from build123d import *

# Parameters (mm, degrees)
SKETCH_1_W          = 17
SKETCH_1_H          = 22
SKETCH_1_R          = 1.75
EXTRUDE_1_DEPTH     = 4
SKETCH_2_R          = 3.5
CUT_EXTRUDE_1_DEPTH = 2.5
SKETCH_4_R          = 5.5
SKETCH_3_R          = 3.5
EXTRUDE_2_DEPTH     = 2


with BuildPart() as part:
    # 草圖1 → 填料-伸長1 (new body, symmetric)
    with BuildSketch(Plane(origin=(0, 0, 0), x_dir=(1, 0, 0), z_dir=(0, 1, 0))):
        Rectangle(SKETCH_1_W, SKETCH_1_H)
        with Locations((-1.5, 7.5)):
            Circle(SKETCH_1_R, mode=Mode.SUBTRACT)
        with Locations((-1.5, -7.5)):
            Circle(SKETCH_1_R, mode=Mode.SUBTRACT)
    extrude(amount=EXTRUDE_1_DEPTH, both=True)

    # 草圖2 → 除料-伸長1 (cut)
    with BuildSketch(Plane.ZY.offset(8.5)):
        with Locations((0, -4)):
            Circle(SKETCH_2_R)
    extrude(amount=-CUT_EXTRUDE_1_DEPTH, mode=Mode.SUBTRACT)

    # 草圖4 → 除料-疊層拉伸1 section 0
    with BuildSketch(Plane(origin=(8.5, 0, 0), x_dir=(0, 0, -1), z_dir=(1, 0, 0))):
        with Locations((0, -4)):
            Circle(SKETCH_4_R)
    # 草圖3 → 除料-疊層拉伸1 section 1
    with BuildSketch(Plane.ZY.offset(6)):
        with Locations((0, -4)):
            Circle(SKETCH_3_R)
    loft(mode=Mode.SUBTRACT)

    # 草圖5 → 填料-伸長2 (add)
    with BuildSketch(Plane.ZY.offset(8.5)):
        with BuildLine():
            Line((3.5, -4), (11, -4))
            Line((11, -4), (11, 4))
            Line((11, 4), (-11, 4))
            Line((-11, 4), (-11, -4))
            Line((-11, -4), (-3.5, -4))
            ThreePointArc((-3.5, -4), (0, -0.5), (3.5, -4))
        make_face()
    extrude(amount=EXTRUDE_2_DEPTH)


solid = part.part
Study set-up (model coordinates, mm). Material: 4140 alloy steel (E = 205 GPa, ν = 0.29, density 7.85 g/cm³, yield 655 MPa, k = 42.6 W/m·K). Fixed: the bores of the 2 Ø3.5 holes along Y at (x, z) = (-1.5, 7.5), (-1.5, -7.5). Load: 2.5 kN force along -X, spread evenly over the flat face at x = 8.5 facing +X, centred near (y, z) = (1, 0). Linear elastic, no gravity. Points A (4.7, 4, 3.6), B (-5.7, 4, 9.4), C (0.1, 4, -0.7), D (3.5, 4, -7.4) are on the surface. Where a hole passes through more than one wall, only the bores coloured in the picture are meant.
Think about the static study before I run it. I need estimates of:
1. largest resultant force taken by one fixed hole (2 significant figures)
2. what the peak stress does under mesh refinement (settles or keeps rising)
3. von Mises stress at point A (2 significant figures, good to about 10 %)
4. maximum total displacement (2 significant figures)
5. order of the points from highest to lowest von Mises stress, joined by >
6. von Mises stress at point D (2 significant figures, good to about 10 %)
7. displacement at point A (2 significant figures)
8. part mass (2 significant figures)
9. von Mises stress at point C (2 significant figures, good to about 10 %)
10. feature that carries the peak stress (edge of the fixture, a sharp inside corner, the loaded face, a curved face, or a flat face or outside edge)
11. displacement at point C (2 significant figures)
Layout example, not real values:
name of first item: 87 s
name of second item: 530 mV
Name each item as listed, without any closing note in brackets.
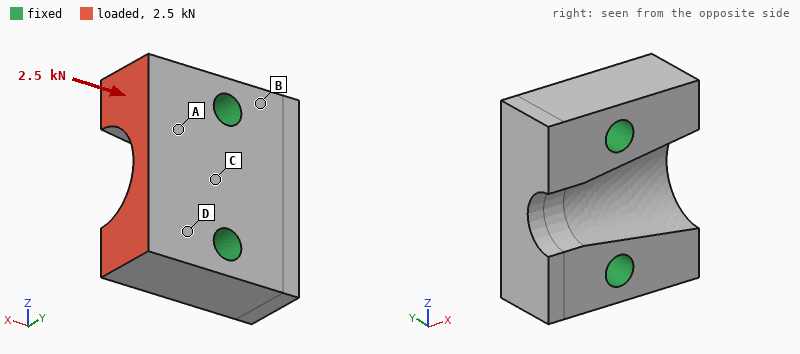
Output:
largest resultant force taken by one fixed hole: 1.3 kN
what the peak stress does under mesh refinement: keeps rising
von Mises stress at point A: 19 MPa
maximum total displacement: 1.2 µm
order of the points from highest to lowest von Mises stress, joined by >: D > A > C > B
von Mises stress at point D: 25 MPa
displacement at point A: 0.75 µm
part mass: 21 g
von Mises stress at point C: 8.7 MPa
feature that carries the peak stress: edge of the fixture
displacement at point C: 0.48 µm
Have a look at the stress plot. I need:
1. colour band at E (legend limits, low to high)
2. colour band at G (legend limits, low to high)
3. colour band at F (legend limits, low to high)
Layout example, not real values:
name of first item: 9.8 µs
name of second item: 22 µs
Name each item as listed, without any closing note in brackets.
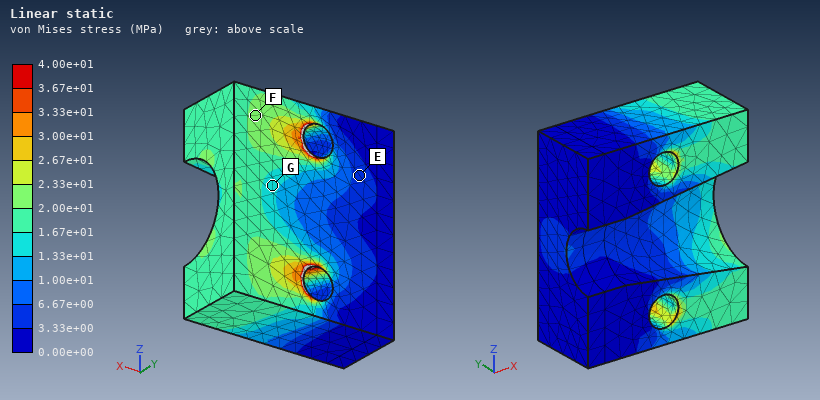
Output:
colour band at E: 3.33e+00 to 6.67e+00 MPa
colour band at G: 1.33e+01 to 1.67e+01 MPa
colour band at F: 2.00e+01 to 2.33e+01 MPa
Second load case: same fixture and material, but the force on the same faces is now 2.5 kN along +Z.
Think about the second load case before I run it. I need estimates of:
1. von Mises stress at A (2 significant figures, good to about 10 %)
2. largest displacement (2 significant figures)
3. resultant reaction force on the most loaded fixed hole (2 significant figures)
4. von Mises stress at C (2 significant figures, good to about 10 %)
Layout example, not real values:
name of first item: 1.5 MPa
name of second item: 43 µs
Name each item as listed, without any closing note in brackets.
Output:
von Mises stress at A: 47 MPa
largest displacement: 6.0 µm
resultant reaction force on the most loaded fixed hole: 1.7 kN
von Mises stress at C: 35 MPa
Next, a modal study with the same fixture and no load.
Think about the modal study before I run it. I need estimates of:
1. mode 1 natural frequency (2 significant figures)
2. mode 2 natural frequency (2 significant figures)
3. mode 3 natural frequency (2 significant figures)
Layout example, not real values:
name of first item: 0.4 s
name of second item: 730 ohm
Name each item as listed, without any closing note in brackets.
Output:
mode 1 natural frequency: 51 kHz
mode 2 natural frequency: 58 kHz
mode 3 natural frequency: 59 kHz
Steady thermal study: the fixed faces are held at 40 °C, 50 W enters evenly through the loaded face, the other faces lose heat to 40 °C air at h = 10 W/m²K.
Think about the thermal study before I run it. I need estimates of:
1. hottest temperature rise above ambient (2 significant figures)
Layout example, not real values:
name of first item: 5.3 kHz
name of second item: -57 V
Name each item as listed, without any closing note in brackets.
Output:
hottest temperature rise above ambient: 80 K
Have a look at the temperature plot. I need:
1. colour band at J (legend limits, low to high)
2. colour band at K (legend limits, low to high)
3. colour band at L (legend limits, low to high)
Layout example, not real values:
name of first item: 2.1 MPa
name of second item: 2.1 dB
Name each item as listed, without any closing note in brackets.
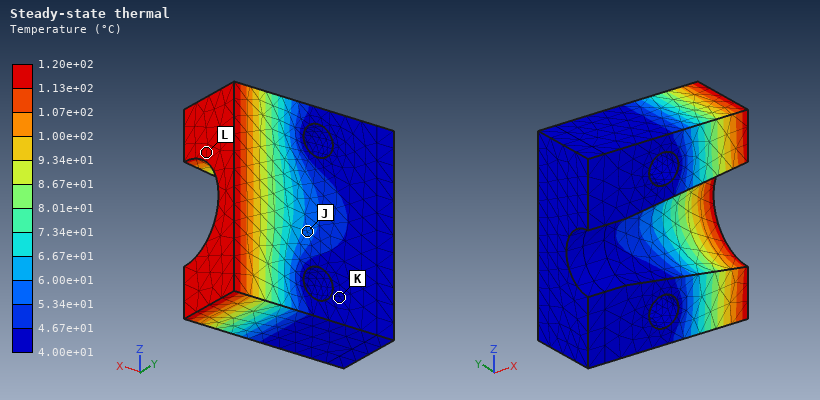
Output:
colour band at J: 5.34e+01 to 6.00e+01 °C
colour band at K: 4.00e+01 to 4.67e+01 °C
colour band at L: 1.13e+02 to 1.20e+02 °C
